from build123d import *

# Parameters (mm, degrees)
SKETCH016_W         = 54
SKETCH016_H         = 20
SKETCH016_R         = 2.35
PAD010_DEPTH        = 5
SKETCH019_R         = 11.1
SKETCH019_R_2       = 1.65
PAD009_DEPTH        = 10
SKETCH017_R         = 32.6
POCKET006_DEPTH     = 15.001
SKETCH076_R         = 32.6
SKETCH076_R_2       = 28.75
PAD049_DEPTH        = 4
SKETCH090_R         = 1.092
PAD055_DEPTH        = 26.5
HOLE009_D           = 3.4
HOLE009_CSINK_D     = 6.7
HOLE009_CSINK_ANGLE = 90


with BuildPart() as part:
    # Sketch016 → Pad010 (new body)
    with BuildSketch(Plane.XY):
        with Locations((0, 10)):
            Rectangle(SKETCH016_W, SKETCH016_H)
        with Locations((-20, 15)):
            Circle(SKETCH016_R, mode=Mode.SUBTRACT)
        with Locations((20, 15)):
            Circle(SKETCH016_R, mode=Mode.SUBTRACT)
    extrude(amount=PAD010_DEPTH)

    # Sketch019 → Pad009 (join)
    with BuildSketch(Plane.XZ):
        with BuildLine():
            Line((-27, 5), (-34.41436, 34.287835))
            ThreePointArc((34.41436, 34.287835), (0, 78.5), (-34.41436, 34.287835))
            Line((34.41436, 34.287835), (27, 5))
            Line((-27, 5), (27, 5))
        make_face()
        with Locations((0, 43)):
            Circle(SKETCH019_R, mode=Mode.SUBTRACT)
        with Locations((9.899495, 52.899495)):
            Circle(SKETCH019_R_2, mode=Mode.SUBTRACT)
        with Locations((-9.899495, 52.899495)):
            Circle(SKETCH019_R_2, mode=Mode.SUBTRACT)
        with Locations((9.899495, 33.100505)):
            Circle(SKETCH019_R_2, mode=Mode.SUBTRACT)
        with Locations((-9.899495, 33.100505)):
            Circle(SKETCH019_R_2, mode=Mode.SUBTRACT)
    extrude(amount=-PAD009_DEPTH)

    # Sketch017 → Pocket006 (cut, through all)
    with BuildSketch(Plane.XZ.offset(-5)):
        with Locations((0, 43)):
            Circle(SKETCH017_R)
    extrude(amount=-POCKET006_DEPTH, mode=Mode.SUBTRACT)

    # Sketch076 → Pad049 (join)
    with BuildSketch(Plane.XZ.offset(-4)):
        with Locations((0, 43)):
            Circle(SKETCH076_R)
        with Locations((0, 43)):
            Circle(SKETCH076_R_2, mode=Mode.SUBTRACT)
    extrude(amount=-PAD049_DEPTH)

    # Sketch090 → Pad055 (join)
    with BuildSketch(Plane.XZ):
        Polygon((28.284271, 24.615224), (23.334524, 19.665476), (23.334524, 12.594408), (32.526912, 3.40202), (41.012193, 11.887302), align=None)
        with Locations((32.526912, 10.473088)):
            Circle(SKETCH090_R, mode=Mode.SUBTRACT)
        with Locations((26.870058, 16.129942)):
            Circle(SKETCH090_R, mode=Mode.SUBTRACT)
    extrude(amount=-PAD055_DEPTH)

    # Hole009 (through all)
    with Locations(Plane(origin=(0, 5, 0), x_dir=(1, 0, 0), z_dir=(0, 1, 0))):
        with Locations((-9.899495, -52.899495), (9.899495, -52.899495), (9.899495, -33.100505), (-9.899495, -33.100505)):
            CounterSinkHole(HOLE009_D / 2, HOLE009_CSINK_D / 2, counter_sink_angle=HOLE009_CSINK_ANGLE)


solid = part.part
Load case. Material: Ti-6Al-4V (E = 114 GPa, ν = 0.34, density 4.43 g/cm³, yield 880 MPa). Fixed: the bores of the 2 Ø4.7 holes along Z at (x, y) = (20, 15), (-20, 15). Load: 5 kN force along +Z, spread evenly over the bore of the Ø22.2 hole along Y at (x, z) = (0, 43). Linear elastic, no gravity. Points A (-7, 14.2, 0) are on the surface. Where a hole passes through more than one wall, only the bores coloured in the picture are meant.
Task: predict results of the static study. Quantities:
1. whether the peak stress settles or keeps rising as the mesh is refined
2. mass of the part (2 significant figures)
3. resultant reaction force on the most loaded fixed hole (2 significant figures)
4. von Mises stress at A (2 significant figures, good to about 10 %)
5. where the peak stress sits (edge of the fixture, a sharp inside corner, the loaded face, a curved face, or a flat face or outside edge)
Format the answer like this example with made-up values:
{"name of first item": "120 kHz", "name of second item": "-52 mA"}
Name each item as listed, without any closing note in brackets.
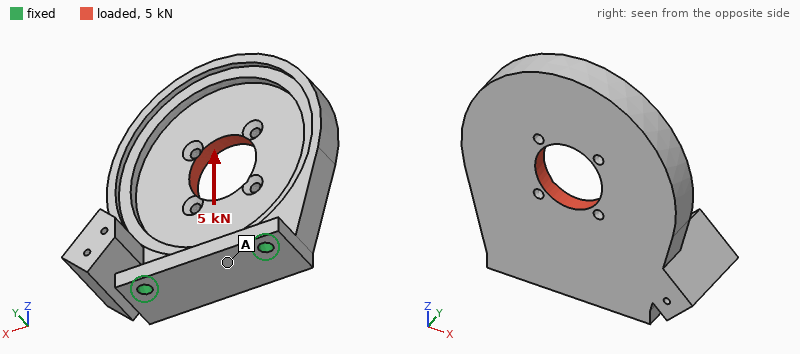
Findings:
{"whether the peak stress settles or keeps rising as the mesh is refined": "keeps rising", "mass of the part": "160 g", "resultant reaction force on the most loaded fixed hole": "2.5 kN", "von Mises stress at A": "62 MPa", "where the peak stress sits": "edge of the fixture"}
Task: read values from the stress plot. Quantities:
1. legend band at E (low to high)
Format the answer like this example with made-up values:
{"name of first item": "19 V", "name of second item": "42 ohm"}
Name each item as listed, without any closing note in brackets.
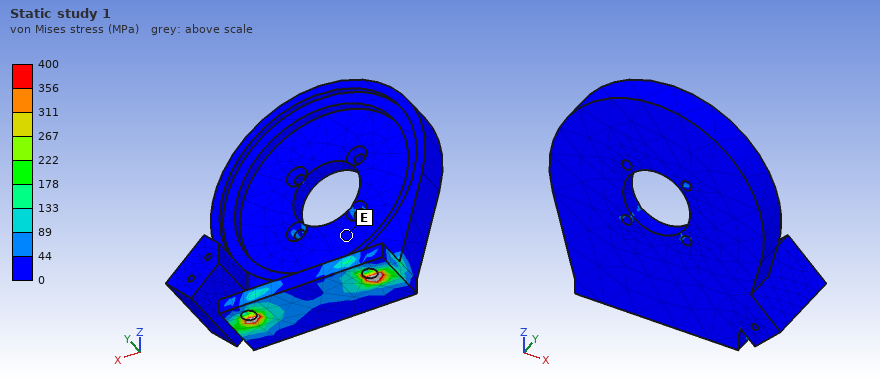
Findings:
{"legend band at E": "0 to 44 MPa"}
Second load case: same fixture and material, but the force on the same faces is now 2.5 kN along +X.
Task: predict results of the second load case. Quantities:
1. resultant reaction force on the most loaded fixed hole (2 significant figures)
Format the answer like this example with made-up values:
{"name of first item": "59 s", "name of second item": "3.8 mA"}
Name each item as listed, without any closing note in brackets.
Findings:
{"resultant reaction force on the most loaded fixed hole": "2.8 kN"}
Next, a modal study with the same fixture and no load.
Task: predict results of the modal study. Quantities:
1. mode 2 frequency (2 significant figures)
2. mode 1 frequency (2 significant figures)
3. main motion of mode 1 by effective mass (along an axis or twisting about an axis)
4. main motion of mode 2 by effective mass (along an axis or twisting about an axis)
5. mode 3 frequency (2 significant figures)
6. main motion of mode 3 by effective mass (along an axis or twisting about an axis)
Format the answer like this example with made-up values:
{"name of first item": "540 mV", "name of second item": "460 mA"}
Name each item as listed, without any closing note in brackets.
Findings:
{"mode 2 frequency": "2200 Hz", "mode 1 frequency": "760 Hz", "main motion of mode 1 by effective mass": "along Y", "main motion of mode 2 by effective mass": "along X", "mode 3 frequency": "3700 Hz", "main motion of mode 3 by effective mass": "along X"}
